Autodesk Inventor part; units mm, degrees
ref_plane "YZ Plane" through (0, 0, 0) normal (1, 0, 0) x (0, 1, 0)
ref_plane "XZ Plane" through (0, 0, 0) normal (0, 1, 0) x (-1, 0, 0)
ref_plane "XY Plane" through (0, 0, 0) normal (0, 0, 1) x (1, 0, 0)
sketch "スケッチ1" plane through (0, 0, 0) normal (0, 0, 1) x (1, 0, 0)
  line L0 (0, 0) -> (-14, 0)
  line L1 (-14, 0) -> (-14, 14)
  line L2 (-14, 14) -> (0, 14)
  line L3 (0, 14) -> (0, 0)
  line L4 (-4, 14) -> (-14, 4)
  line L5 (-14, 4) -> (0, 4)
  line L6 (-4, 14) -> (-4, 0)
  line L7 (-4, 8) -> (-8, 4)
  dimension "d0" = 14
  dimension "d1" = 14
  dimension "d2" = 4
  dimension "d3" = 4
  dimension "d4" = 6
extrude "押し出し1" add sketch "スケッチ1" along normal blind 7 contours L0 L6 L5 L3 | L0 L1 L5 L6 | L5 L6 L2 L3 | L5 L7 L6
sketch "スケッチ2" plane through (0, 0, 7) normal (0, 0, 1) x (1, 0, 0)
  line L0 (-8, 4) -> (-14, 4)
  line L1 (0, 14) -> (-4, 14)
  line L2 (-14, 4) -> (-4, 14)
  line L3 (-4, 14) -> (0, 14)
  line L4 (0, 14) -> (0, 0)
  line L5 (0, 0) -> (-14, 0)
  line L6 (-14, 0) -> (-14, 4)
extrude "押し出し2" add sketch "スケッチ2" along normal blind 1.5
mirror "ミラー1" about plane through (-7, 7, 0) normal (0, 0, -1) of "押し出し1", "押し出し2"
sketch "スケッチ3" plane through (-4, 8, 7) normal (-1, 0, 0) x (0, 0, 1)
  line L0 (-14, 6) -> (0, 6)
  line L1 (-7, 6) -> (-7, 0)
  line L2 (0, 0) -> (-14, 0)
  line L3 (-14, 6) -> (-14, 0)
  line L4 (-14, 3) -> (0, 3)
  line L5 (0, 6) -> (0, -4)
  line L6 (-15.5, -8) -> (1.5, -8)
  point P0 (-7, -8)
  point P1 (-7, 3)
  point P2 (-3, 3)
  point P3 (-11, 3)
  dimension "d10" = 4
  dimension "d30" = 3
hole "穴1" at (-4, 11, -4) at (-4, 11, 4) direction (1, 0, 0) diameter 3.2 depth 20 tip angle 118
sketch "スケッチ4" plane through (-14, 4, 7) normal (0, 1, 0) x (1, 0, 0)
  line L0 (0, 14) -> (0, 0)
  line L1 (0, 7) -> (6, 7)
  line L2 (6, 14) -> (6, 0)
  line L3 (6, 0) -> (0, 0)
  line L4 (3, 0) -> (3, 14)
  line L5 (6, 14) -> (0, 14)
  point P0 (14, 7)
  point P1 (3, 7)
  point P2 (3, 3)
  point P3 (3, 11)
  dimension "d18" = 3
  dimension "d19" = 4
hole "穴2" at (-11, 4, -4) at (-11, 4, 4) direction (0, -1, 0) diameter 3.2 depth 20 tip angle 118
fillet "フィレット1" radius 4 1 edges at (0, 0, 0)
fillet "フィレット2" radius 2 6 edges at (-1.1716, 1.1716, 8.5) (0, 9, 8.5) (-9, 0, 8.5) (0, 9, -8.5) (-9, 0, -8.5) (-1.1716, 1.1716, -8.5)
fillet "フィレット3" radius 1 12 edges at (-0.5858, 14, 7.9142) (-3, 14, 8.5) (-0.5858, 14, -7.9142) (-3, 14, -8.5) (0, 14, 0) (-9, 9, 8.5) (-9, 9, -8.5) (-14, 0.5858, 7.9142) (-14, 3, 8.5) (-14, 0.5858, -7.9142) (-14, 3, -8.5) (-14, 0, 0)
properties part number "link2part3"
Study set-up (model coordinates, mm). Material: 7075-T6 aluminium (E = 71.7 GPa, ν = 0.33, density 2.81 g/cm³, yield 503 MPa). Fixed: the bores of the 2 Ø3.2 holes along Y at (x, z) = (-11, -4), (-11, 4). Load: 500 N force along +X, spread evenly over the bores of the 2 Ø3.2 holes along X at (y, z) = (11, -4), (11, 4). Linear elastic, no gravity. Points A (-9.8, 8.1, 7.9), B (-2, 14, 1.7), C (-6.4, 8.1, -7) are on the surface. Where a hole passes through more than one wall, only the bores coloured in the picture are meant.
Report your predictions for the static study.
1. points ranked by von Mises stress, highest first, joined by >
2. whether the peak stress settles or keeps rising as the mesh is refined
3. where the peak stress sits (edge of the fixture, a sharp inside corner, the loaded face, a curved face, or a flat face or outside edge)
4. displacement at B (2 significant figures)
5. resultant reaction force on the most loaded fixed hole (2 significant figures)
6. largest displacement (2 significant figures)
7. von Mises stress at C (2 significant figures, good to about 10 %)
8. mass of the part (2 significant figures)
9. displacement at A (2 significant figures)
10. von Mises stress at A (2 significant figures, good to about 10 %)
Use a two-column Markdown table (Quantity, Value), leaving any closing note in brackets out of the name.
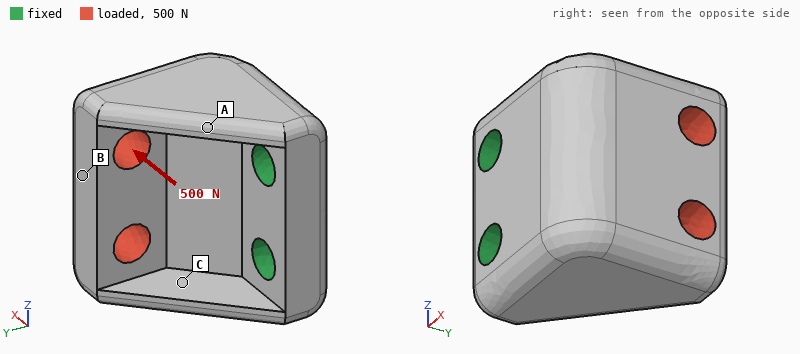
| Quantity | Value |
|---|---|
| points ranked by von Mises stress, highest first, joined by > | A > C > B |
| whether the peak stress settles or keeps rising as the mesh is refined | keeps rising |
| where the peak stress sits | edge of the fixture |
| displacement at B | 36 µm |
| resultant reaction force on the most loaded fixed hole | 250 N |
| largest displacement | 38 µm |
| von Mises stress at C | 29 MPa |
| mass of the part | 4.6 g |
| displacement at A | 12 µm |
| von Mises stress at A | 49 MPa |
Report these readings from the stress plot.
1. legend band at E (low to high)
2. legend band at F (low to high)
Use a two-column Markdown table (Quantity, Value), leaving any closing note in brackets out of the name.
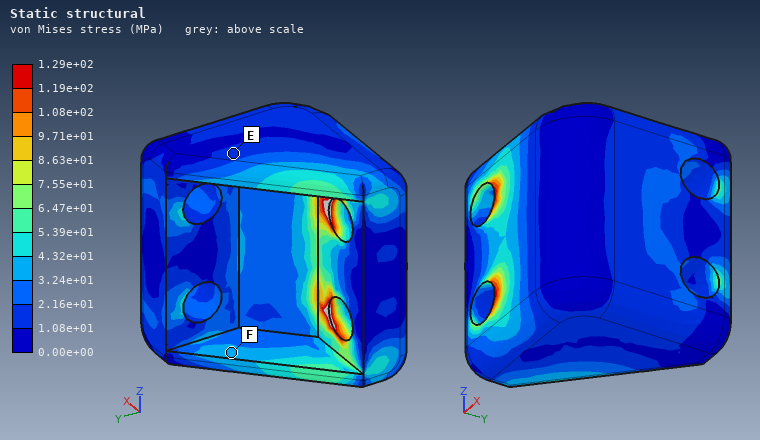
| Quantity | Value |
|---|---|
| legend band at E | 1.08e+01 to 2.16e+01 MPa |
| legend band at F | 3.24e+01 to 4.32e+01 MPa |
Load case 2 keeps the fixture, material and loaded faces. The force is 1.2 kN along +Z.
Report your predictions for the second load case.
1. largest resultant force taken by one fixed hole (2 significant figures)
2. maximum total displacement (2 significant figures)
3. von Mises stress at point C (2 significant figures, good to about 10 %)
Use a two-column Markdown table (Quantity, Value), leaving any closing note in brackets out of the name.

| Quantity | Value |
|---|---|
| largest resultant force taken by one fixed hole | 1.4 kN |
| maximum total displacement | 48 µm |
| von Mises stress at point C | 35 MPa |
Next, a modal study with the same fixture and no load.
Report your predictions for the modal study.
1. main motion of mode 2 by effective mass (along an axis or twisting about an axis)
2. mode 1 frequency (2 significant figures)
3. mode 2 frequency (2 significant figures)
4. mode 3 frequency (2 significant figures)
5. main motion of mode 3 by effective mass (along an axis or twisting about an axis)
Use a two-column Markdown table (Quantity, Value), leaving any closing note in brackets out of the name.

| Quantity | Value |
|---|---|
| main motion of mode 2 by effective mass | along Z |
| mode 1 frequency | 15 kHz |
| mode 2 frequency | 22 kHz |
| mode 3 frequency | 35 kHz |
| main motion of mode 3 by effective mass | along Z |
